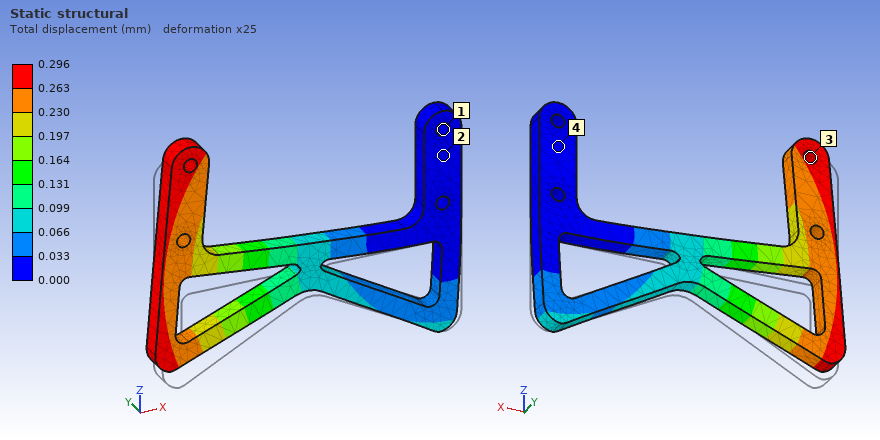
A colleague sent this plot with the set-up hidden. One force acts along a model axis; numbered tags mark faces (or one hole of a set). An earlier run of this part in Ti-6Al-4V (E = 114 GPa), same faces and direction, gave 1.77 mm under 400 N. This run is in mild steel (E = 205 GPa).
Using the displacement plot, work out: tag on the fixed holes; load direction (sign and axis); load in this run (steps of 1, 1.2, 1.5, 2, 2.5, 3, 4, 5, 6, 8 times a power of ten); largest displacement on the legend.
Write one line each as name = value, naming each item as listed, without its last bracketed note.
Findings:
tag on the fixed holes = 1
load direction = +Z
load in this run = 120 N
largest displacement on the legend = 0.296 mm
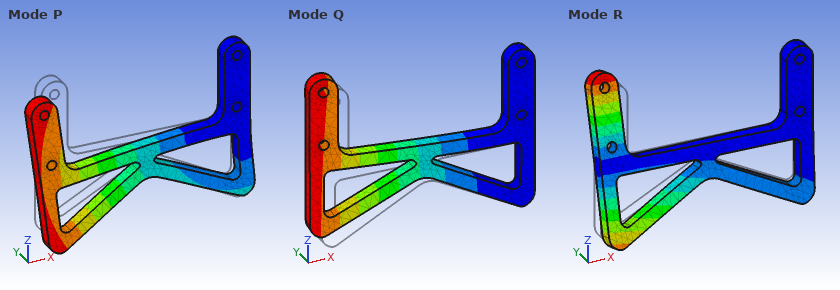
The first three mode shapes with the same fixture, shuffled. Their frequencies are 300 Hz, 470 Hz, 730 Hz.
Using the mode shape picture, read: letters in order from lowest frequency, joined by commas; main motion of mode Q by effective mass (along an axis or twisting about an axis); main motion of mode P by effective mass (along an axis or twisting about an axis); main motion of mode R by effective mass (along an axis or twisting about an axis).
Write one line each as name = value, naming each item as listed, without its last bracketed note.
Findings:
letters in order from lowest frequency, joined by commas = Q, P, R
main motion of mode Q by effective mass = along Y
main motion of mode P by effective mass = along Z
main motion of mode R by effective mass = twisting about X
